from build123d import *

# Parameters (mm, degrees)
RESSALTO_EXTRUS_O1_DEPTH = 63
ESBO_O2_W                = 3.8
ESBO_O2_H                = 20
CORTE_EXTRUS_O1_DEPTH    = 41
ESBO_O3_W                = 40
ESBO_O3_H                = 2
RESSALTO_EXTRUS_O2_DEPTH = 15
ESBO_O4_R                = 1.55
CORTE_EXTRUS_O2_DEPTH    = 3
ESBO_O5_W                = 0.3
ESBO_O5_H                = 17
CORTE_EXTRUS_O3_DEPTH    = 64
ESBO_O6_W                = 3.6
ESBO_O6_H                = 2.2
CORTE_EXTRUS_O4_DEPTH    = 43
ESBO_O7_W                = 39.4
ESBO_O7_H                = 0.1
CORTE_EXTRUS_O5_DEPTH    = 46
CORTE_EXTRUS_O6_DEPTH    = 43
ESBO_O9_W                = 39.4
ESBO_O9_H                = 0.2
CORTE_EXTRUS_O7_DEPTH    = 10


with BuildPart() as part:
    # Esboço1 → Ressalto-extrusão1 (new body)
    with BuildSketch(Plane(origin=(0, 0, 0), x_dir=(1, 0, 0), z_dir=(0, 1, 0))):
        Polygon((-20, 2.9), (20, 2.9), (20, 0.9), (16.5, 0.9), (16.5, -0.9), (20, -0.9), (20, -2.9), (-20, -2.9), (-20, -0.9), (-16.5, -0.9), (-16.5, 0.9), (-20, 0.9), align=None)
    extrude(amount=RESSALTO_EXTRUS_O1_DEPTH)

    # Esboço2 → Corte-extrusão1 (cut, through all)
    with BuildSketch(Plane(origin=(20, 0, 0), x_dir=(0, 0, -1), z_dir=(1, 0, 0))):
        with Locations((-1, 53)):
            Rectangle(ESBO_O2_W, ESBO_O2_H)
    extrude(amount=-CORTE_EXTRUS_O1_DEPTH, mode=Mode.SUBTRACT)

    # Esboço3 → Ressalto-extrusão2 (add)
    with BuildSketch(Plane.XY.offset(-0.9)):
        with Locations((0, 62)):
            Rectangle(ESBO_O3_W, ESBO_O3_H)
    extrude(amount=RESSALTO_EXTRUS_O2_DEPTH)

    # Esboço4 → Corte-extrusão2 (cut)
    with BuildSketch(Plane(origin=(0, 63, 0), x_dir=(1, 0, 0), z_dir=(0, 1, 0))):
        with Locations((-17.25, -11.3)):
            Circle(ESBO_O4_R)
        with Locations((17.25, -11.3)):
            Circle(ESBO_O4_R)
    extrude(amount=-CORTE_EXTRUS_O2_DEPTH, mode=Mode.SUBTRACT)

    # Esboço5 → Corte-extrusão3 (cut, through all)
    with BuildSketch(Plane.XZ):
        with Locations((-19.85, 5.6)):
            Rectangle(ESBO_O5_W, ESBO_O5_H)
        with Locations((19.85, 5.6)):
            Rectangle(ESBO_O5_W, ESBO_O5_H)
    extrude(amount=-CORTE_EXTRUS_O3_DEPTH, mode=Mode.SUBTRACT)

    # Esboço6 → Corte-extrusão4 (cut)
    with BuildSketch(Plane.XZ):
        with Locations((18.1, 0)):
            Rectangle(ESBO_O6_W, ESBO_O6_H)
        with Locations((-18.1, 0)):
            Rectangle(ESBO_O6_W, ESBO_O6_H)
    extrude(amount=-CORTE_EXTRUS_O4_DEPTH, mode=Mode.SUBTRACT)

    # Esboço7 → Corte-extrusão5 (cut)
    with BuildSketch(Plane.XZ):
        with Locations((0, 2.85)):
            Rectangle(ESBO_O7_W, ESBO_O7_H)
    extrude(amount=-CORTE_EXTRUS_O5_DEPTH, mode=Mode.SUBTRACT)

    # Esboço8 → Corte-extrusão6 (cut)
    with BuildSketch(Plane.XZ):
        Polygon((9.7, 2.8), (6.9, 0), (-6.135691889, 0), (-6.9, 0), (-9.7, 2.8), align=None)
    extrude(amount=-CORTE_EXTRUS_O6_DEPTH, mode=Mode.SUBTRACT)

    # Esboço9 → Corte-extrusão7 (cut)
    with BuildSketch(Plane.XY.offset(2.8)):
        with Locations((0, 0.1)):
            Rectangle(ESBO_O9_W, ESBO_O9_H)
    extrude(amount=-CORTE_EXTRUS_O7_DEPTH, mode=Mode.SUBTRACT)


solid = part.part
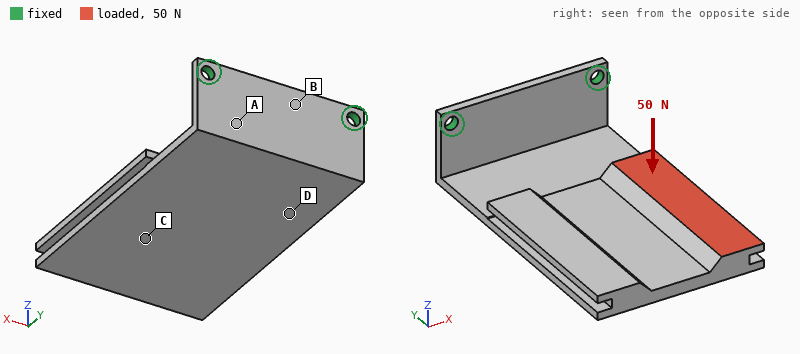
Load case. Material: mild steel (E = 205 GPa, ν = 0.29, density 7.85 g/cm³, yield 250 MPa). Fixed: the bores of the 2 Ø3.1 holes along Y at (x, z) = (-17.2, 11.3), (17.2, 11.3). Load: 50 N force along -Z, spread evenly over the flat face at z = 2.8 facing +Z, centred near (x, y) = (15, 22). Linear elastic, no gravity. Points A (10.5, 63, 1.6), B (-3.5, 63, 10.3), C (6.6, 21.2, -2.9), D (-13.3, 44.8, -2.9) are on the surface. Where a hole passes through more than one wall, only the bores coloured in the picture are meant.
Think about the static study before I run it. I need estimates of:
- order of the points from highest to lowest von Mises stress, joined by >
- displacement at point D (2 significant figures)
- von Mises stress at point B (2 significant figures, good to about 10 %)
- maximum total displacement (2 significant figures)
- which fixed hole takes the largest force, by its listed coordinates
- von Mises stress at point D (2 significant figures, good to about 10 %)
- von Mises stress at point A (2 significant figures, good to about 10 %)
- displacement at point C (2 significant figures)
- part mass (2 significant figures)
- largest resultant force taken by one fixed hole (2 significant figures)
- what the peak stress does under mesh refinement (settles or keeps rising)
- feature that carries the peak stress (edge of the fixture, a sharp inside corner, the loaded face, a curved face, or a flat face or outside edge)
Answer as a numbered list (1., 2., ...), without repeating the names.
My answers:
1. A > D > B > C
2. 0.14 mm
3. 30 MPa
4. 0.67 mm
5. (17.2, 11.3)
6. 55 MPa
7. 75 MPa
8. 0.42 mm
9. 76 g
10. 52 N
11. keeps rising
12. edge of the fixture
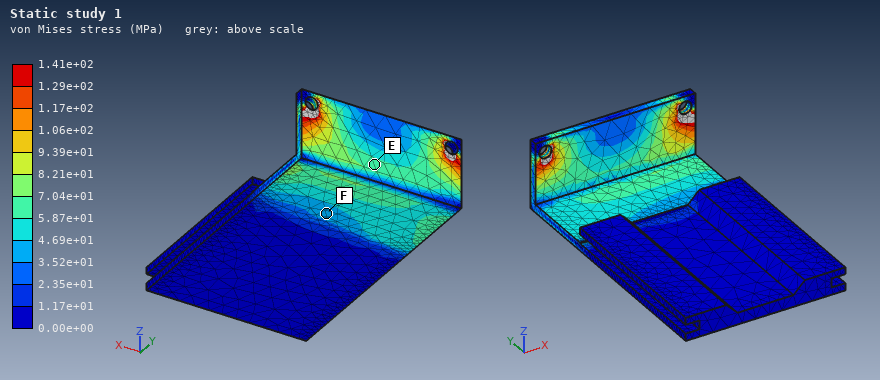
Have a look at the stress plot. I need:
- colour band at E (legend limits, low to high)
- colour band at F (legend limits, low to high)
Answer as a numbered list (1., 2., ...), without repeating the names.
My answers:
1. 5.87e+01 to 7.04e+01 MPa
2. 3.52e+01 to 4.69e+01 MPa
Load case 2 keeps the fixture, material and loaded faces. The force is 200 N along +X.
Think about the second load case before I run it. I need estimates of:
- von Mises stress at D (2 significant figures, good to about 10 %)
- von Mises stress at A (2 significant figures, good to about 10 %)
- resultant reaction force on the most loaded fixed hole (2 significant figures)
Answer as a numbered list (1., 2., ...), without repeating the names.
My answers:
1. 35 MPa
2. 97 MPa
3. 270 N
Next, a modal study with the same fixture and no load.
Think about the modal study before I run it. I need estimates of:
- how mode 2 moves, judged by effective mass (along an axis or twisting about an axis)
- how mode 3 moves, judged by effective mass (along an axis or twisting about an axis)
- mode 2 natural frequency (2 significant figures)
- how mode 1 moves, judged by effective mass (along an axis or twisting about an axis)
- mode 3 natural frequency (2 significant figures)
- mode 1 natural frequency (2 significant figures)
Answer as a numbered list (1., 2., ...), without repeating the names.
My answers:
1. along X
2. along Y
3. 730 Hz
4. along Z
5. 1600 Hz
6. 230 Hz
